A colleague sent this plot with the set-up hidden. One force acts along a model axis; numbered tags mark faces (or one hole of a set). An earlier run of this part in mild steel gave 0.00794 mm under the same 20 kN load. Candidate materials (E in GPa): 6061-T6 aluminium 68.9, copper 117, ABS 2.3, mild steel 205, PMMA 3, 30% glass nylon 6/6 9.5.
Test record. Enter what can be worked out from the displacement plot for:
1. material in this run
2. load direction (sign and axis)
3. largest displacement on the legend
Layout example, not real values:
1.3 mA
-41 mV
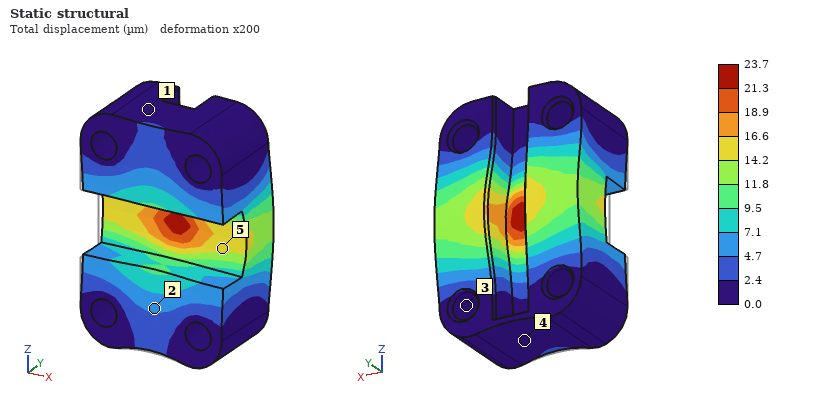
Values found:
6061-T6 aluminium
+Y
23.7 µm
